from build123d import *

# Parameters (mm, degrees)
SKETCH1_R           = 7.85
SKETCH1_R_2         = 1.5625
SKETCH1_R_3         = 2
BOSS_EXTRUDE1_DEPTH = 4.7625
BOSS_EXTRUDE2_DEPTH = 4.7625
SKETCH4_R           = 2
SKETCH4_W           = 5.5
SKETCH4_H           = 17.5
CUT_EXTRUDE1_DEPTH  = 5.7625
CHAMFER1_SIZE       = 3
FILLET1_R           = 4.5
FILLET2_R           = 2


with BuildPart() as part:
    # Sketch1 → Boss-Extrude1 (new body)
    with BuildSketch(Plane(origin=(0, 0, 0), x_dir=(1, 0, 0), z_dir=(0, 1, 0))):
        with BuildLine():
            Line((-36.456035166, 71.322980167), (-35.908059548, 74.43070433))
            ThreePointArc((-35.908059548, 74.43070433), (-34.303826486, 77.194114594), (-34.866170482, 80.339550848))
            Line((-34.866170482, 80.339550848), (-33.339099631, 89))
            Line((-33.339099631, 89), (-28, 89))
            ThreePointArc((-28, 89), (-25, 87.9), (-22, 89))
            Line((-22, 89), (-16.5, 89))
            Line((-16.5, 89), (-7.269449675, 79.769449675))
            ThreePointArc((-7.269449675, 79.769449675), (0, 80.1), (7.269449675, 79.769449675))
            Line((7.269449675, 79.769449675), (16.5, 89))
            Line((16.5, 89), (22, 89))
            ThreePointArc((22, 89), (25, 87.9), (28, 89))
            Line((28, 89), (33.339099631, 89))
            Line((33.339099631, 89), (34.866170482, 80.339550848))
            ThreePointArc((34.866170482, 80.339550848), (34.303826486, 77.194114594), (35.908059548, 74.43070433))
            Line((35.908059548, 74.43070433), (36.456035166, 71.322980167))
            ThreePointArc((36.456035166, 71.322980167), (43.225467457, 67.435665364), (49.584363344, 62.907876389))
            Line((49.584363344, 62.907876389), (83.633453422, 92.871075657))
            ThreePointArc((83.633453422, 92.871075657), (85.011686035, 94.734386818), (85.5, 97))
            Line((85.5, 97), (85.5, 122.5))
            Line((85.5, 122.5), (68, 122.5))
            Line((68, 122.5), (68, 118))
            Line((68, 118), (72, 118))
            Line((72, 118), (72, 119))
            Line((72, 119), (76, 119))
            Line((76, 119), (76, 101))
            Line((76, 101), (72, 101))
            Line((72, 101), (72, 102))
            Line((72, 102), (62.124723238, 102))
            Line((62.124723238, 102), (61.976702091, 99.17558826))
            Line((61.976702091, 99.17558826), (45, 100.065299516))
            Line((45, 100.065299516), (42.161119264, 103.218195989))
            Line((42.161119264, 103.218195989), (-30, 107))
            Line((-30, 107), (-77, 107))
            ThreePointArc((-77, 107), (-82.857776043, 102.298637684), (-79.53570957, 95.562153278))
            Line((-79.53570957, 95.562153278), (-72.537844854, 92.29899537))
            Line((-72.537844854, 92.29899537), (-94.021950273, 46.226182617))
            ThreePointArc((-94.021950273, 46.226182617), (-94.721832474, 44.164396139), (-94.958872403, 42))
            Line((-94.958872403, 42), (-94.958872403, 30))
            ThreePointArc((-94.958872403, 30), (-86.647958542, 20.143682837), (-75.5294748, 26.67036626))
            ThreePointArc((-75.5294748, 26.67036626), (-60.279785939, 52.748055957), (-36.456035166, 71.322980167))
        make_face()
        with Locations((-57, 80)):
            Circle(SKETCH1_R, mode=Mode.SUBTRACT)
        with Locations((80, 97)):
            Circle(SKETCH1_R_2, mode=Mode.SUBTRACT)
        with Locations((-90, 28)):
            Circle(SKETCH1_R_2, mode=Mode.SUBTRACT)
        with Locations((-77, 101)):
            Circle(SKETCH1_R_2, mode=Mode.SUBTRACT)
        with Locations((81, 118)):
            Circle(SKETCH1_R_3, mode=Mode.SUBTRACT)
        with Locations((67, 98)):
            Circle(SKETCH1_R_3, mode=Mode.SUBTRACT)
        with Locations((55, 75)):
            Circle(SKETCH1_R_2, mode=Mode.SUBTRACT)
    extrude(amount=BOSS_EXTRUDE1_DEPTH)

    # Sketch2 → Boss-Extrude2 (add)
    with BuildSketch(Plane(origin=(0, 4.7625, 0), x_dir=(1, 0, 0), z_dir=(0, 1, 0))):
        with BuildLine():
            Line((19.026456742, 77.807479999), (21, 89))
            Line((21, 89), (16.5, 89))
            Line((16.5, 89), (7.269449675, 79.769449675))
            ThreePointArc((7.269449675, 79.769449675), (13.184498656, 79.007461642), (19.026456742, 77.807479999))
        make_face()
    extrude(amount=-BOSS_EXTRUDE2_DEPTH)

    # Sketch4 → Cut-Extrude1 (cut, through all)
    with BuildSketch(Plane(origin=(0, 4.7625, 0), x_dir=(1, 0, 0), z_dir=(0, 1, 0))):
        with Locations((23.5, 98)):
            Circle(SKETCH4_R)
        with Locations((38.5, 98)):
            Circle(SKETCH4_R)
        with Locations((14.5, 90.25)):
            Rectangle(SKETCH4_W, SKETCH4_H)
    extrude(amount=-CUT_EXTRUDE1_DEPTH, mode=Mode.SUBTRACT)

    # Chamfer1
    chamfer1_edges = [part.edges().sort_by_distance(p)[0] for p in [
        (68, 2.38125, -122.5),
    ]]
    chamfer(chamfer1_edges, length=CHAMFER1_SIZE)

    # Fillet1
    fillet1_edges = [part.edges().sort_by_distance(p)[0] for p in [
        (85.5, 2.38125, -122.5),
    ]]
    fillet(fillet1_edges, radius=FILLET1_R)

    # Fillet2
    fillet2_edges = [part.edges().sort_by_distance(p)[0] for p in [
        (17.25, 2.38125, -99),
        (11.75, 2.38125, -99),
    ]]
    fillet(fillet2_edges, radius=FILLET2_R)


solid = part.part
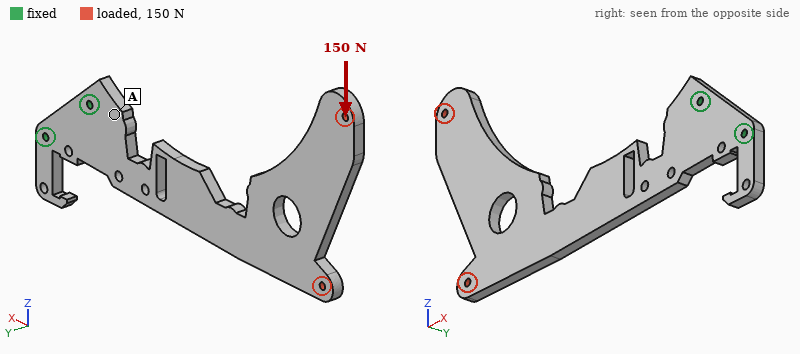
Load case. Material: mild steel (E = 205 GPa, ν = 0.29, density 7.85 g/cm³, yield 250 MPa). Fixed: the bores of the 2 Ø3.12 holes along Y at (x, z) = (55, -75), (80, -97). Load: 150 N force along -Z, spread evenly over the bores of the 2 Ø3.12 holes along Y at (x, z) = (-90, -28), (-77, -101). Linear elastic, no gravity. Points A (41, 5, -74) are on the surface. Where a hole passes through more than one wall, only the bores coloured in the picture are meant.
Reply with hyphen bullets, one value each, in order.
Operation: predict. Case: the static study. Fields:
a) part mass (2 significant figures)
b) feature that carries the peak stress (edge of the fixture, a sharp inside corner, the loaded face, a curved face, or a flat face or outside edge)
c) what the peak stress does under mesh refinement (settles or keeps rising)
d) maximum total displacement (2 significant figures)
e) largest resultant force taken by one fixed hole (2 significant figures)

- 210 g
- a sharp inside corner
- keeps rising
- 0.60 mm
- 780 N
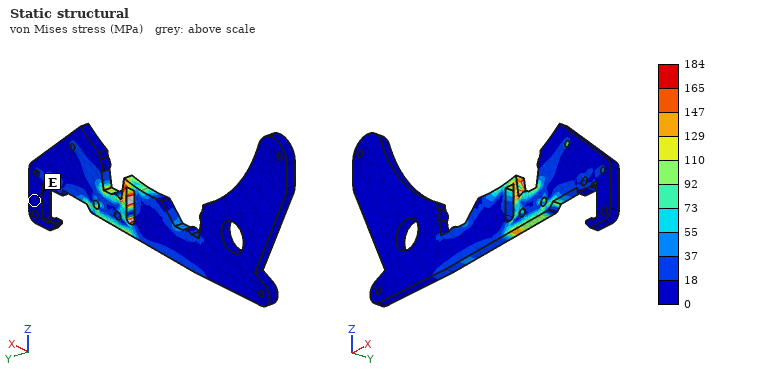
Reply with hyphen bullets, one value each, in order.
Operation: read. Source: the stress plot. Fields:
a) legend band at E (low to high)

- 0 to 18 MPa
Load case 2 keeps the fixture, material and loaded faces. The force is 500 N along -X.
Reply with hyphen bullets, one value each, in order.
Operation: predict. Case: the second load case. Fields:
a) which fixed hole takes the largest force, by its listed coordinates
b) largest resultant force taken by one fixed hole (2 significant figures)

- (55, -75)
- 630 N
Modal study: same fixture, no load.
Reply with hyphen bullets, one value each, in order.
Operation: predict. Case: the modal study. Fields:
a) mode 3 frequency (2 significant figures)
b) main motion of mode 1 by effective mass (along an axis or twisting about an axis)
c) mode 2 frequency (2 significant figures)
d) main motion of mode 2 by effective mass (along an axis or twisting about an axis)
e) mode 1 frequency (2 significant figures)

- 390 Hz
- along Y
- 300 Hz
- along Z
- 96 Hz
